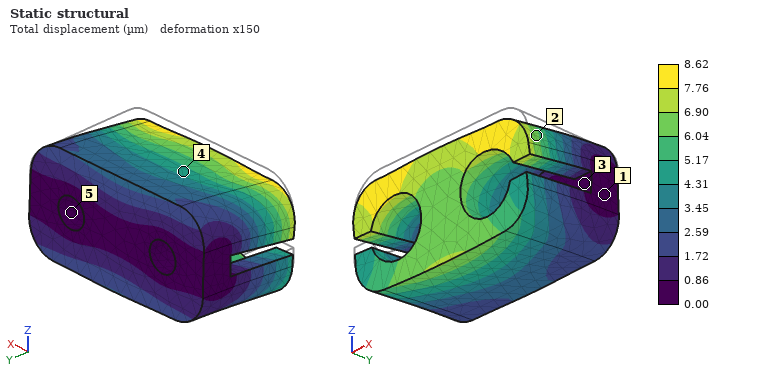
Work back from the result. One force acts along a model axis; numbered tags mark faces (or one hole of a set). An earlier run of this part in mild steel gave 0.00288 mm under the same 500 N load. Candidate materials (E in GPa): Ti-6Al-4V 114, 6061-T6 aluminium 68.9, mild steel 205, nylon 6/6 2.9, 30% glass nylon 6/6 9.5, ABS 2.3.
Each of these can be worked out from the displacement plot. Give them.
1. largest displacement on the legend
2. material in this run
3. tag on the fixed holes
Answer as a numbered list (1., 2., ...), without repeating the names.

1. 8.62 µm
2. 6061-T6 aluminium
3. 5
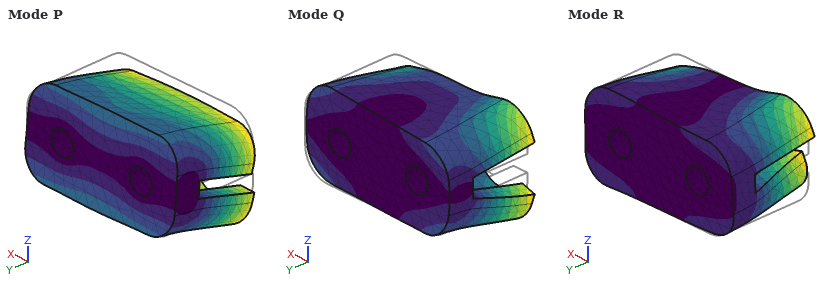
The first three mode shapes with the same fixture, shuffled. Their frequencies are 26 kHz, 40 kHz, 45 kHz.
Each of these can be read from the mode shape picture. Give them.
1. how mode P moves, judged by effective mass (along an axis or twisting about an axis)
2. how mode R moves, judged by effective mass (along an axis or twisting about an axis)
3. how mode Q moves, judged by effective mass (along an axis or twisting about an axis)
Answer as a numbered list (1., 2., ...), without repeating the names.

1. along Z
2. twisting about Y
3. along X
